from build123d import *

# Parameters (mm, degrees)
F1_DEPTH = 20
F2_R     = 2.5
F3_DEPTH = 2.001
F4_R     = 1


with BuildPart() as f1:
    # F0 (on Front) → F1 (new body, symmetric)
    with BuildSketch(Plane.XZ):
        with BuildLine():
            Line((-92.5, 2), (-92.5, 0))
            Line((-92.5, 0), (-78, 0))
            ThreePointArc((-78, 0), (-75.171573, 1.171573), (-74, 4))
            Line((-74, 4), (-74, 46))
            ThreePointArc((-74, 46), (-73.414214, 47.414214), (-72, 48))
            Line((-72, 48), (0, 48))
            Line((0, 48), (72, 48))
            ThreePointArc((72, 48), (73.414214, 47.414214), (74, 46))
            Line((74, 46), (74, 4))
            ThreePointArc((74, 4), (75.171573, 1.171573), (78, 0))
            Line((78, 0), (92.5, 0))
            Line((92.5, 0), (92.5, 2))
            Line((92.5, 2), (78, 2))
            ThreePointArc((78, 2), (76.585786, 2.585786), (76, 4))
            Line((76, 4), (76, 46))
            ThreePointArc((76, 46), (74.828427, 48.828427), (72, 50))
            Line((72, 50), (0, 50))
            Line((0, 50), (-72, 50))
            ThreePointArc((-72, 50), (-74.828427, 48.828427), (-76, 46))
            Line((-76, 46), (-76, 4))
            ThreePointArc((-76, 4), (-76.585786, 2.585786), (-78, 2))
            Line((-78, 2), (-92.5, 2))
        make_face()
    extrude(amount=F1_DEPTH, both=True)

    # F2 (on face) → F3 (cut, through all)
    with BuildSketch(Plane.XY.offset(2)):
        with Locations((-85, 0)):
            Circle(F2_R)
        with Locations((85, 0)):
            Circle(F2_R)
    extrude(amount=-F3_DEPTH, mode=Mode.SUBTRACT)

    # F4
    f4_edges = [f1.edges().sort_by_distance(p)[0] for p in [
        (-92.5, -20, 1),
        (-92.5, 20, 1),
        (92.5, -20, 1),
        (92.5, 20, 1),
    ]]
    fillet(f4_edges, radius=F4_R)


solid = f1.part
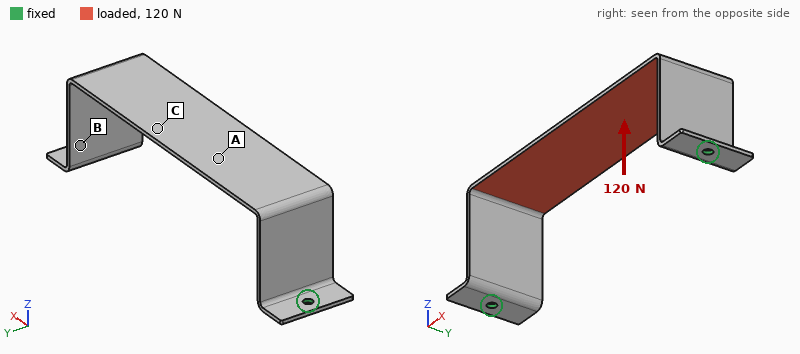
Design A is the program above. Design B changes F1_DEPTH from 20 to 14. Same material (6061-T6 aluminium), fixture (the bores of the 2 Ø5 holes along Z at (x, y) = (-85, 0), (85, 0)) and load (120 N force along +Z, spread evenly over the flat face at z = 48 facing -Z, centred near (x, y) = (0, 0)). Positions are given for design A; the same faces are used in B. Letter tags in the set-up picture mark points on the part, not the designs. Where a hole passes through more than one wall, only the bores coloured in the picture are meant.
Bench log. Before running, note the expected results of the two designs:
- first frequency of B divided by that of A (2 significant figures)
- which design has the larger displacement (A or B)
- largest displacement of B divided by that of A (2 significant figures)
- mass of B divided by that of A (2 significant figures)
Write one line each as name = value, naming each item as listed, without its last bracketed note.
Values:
first frequency of B divided by that of A = 1.0
which design has the larger displacement = B
largest displacement of B divided by that of A = 1.4
mass of B divided by that of A = 0.70
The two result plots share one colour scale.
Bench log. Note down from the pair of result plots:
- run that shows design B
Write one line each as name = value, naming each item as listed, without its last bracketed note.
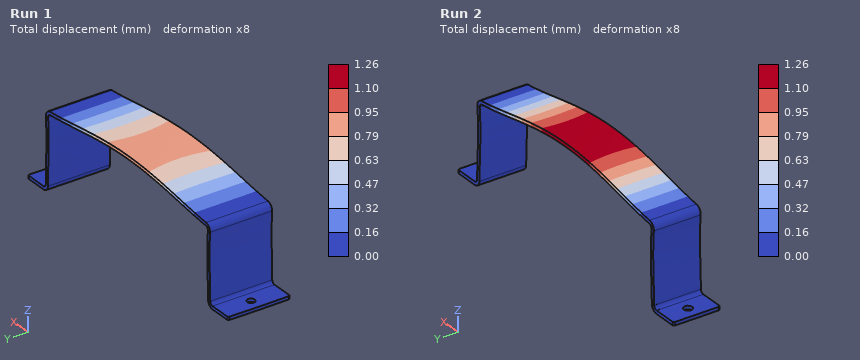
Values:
run that shows design B = Run 2
